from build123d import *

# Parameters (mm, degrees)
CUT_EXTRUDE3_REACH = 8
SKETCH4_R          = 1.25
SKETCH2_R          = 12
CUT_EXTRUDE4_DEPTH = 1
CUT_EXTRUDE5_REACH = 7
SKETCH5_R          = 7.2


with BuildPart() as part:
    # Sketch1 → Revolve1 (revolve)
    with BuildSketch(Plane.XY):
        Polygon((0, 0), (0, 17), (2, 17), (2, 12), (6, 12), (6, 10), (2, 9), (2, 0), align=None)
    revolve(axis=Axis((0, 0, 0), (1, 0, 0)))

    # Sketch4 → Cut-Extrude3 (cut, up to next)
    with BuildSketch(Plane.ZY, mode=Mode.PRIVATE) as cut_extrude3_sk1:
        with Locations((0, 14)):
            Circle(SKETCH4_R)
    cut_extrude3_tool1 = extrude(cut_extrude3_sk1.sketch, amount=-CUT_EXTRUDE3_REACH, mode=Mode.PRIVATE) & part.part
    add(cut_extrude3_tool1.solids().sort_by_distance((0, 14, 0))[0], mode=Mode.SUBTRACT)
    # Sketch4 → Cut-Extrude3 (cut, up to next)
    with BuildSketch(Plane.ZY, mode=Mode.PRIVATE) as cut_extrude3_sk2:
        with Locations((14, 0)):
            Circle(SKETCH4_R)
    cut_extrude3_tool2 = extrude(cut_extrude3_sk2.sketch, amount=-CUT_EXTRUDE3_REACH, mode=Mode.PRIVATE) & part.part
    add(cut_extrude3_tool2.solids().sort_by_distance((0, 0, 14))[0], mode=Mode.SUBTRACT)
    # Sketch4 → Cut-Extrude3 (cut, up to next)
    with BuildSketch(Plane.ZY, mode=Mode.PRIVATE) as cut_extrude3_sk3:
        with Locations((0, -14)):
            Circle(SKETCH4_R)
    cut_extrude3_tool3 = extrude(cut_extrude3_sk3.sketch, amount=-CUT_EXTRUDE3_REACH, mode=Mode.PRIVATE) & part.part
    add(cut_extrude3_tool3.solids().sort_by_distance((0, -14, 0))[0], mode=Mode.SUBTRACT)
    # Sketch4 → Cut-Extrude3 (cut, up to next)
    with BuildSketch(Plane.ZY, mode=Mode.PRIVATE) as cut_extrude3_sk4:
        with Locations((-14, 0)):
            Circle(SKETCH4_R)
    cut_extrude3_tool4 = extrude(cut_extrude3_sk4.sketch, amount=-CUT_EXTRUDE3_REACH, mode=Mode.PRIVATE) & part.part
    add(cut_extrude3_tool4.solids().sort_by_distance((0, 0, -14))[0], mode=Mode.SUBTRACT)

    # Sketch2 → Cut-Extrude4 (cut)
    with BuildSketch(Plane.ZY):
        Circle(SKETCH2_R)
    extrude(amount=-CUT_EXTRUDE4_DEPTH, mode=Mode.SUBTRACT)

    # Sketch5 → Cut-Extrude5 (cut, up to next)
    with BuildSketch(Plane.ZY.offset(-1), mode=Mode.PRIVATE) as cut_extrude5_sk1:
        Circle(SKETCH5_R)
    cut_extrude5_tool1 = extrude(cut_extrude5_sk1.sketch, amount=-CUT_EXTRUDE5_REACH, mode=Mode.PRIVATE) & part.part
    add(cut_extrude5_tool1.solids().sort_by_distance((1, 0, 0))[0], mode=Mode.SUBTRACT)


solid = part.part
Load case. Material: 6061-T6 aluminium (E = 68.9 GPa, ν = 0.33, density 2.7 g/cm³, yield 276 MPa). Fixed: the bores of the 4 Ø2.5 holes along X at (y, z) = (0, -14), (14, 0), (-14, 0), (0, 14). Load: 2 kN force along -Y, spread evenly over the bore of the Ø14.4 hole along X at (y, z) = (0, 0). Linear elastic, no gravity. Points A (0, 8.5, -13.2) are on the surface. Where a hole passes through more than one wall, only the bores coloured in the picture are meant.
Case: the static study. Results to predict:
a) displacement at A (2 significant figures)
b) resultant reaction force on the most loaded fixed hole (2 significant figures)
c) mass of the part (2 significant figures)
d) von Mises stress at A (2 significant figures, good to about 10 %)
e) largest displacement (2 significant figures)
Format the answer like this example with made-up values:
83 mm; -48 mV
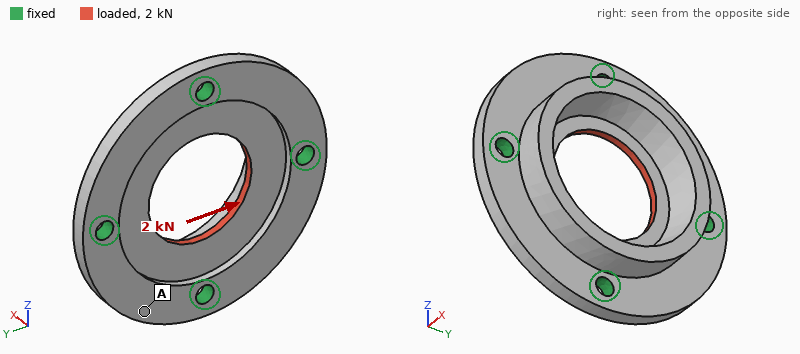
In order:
2.8 µm; 500 N; 5.0 g; 16 MPa; 7.7 µm
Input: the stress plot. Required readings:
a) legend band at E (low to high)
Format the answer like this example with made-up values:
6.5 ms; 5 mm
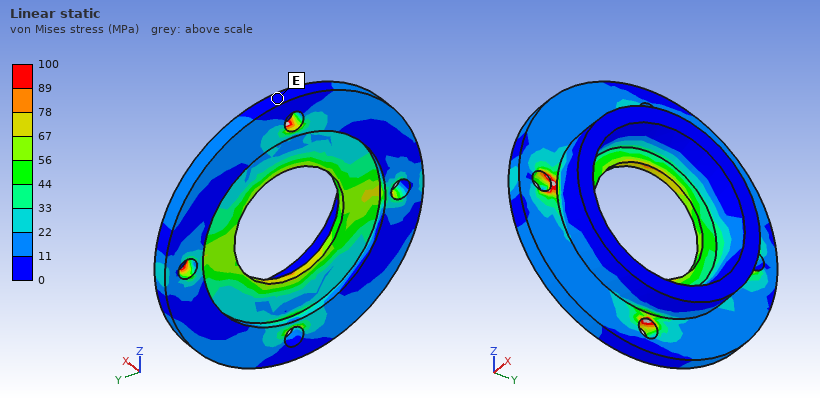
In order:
0 to 11 MPa
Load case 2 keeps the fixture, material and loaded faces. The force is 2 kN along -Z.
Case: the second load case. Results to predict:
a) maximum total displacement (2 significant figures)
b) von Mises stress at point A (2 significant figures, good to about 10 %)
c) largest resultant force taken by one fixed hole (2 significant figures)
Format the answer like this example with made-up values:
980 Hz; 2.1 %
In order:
7.7 µm; 10 MPa; 500 N
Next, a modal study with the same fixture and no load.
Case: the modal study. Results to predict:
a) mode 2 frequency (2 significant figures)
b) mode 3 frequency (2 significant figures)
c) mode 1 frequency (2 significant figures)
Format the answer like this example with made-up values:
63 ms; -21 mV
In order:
26 kHz; 26 kHz; 23 kHz
